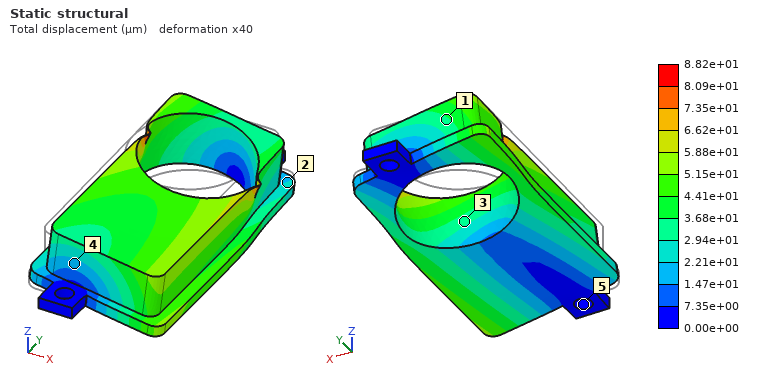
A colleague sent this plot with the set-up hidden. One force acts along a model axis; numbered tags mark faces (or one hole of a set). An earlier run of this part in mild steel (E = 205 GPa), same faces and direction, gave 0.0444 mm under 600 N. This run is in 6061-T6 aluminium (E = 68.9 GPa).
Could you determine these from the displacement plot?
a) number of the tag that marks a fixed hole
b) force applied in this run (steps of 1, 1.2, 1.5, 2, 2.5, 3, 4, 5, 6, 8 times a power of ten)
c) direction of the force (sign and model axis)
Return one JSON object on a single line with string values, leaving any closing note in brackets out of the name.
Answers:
{"number of the tag that marks a fixed hole": "5", "force applied in this run": "400 N", "direction of the force": "+X"}
